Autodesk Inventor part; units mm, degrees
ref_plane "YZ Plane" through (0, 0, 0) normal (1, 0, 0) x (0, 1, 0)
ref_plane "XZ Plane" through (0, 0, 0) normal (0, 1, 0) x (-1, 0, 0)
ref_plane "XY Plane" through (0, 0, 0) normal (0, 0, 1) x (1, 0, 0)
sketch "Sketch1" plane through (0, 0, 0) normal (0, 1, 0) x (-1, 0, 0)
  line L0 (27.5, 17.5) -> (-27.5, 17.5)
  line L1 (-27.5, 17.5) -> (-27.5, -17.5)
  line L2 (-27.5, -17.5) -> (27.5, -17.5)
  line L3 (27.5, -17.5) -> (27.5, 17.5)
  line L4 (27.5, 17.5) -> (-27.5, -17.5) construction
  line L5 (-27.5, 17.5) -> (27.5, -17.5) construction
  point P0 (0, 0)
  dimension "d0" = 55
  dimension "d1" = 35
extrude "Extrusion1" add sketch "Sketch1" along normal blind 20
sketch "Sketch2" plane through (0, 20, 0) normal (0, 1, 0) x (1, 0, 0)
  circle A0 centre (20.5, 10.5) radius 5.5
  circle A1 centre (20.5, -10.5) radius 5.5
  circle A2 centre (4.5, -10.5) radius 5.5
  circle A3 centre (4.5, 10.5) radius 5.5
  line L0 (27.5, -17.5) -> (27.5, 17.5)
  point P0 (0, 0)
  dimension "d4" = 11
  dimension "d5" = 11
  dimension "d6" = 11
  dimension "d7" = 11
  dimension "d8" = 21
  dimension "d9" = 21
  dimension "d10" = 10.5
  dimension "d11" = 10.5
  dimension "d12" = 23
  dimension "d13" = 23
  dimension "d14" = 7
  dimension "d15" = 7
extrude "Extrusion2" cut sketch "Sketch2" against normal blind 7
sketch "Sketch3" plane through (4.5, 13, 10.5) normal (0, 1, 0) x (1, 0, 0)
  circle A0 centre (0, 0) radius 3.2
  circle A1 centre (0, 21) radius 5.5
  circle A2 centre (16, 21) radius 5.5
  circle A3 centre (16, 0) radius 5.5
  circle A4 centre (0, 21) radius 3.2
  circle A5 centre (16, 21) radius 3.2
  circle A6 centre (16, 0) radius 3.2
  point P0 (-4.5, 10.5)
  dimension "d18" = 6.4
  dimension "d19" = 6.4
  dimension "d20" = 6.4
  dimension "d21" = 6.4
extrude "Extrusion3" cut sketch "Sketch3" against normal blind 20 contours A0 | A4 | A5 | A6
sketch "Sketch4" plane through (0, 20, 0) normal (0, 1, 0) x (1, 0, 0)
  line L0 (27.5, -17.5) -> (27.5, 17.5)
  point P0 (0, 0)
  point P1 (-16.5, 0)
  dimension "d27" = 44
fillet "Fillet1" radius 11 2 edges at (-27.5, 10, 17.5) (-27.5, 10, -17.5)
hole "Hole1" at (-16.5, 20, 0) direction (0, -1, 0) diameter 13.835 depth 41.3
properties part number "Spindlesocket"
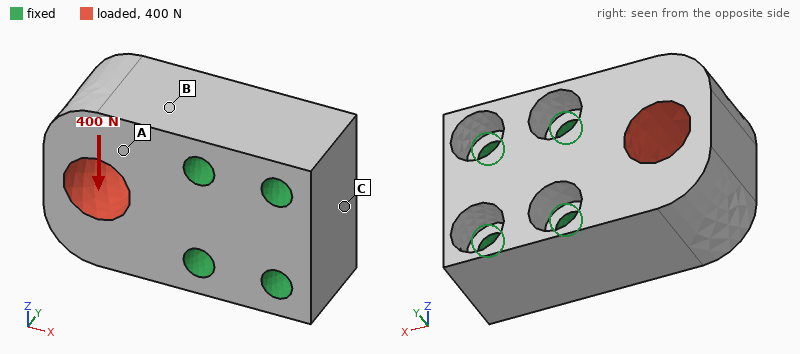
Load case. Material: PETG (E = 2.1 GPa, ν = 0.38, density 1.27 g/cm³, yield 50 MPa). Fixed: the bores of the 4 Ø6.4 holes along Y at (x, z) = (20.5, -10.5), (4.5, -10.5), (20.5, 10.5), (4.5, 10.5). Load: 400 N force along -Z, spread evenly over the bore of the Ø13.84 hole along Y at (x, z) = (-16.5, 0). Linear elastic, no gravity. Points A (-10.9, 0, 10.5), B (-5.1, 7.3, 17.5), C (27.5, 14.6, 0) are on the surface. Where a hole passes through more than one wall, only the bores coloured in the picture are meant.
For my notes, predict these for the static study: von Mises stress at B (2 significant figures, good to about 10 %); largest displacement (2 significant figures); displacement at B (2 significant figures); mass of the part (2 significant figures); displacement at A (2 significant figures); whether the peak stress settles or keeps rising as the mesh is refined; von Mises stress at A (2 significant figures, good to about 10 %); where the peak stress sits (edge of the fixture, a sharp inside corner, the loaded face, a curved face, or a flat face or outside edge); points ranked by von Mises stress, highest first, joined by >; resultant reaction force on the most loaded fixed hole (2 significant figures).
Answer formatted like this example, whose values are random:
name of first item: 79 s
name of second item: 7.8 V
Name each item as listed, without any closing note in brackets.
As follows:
von Mises stress at B: 1.7 MPa
largest displacement: 61 µm
displacement at B: 19 µm
mass of the part: 38 g
displacement at A: 22 µm
whether the peak stress settles or keeps rising as the mesh is refined: keeps rising
von Mises stress at A: 1.4 MPa
where the peak stress sits: edge of the fixture
points ranked by von Mises stress, highest first, joined by >: B > A > C
resultant reaction force on the most loaded fixed hole: 350 N
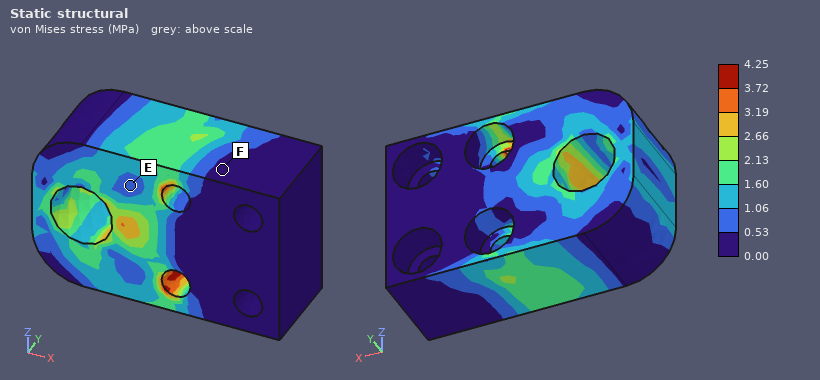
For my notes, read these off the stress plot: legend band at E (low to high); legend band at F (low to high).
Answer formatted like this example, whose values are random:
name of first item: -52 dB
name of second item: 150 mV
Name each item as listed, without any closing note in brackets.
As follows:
legend band at E: 0.53 to 1.06 MPa
legend band at F: 0.00 to 0.53 MPa
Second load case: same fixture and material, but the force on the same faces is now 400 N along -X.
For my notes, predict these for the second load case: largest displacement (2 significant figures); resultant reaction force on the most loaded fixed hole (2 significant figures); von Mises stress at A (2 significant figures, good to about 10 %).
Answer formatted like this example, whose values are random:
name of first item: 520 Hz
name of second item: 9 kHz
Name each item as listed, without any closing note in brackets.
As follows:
largest displacement: 27 µm
resultant reaction force on the most loaded fixed hole: 170 N
von Mises stress at A: 0.92 MPa
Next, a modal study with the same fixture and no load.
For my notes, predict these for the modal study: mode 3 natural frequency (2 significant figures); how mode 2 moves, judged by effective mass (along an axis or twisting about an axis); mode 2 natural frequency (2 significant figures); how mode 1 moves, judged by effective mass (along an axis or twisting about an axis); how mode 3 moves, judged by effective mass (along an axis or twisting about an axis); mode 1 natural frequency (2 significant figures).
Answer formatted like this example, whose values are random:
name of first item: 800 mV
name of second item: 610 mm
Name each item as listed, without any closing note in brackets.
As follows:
mode 3 natural frequency: 4900 Hz
how mode 2 moves, judged by effective mass: along Z
mode 2 natural frequency: 4000 Hz
how mode 1 moves, judged by effective mass: along Y
how mode 3 moves, judged by effective mass: twisting about X
mode 1 natural frequency: 2900 Hz
